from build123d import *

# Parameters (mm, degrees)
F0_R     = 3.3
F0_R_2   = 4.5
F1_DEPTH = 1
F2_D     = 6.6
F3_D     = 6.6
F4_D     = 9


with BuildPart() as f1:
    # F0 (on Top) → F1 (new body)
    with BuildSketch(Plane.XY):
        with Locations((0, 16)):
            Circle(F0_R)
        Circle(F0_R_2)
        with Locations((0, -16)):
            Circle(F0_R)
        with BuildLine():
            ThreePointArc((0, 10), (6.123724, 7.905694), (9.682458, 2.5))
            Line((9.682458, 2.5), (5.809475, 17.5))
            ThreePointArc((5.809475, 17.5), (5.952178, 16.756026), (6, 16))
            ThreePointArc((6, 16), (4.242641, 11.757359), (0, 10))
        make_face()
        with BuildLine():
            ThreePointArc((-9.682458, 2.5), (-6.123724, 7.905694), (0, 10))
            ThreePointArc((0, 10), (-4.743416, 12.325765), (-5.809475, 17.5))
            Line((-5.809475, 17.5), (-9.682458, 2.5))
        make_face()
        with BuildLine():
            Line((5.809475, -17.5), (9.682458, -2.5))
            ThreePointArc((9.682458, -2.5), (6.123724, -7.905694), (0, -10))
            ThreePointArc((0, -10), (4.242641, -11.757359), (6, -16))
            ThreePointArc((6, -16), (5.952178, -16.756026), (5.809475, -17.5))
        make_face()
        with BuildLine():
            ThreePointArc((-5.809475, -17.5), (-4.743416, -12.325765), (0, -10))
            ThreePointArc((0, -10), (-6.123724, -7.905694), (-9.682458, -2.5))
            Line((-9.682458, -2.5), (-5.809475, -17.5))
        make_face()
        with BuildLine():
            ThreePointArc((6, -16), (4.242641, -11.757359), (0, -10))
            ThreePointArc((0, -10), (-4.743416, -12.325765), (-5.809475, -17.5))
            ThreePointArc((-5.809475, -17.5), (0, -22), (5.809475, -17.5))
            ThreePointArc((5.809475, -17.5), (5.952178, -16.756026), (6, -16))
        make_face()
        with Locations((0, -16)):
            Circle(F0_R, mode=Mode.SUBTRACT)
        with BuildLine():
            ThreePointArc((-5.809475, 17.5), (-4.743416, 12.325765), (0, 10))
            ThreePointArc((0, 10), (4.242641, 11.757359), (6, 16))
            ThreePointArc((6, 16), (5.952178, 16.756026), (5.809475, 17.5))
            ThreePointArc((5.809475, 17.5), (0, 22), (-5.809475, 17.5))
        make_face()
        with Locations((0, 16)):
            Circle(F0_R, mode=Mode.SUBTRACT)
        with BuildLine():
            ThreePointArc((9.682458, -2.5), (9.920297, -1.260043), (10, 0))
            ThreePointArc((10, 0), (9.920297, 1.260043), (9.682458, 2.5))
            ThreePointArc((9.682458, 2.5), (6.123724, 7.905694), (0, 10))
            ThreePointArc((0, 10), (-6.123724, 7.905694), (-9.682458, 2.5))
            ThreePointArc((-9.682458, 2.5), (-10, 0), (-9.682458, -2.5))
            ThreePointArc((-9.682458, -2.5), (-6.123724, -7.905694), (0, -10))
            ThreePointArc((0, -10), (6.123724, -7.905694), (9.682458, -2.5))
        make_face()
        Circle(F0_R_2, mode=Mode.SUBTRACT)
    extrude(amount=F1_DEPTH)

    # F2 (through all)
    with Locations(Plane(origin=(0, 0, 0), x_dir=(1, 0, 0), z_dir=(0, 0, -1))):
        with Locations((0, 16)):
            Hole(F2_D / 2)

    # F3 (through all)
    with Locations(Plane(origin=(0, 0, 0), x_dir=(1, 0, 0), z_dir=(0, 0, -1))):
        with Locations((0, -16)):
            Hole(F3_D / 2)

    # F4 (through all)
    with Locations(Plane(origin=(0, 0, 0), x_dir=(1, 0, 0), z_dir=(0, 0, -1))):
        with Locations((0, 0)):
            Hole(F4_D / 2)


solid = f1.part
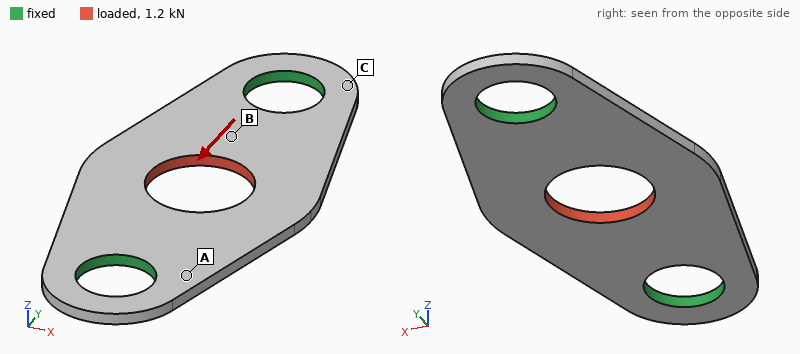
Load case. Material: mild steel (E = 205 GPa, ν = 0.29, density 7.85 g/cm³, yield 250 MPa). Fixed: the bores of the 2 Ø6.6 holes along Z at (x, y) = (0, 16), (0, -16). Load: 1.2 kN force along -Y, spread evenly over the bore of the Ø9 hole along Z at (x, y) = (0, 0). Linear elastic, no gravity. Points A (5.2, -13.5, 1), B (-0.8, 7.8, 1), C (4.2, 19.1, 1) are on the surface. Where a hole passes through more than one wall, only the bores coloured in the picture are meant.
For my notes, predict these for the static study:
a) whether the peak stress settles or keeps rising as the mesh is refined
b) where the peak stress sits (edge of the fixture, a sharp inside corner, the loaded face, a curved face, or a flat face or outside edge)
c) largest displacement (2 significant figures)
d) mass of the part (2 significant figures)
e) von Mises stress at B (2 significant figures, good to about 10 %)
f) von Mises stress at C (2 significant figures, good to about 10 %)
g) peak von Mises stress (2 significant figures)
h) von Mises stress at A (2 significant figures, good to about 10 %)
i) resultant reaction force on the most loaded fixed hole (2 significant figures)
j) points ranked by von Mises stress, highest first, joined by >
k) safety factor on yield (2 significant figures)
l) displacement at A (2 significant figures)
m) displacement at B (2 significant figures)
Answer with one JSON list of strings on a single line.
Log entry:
["settles", "the loaded face", "3.2 µm", "4.0 g", "55 MPa", "11 MPa", "77 MPa", "29 MPa", "600 N", "B > A > C", "3.2", "0.77 µm", "1.4 µm"]
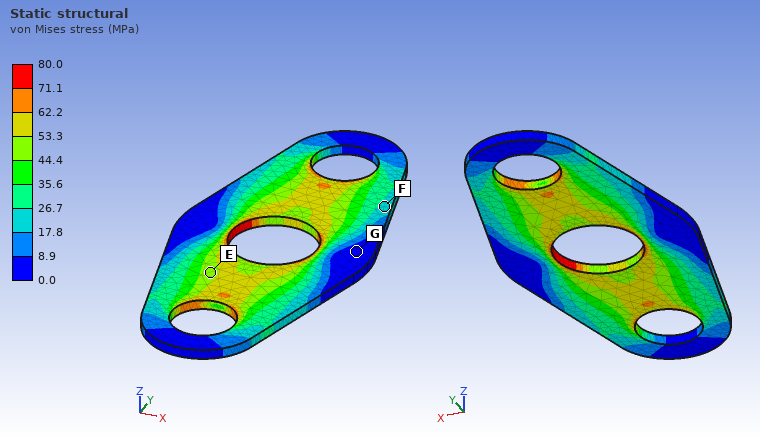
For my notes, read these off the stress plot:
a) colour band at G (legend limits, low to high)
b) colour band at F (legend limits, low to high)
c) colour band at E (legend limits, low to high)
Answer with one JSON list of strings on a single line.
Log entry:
["0.0 to 8.9 MPa", "17.8 to 26.7 MPa", "44.4 to 53.3 MPa"]
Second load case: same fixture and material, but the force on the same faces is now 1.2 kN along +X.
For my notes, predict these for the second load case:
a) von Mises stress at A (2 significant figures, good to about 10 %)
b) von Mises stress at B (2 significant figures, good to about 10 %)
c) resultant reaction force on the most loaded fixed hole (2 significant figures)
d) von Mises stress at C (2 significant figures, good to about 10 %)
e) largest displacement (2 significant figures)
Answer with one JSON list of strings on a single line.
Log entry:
["38 MPa", "83 MPa", "600 N", "15 MPa", "8.9 µm"]
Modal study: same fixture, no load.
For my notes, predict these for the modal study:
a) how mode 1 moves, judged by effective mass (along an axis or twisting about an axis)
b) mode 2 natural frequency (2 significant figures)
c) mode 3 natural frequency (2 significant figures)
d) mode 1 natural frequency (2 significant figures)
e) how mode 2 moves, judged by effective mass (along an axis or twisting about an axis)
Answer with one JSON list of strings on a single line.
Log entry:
["along Z", "6800 Hz", "16 kHz", "6400 Hz", "twisting about Y"]
